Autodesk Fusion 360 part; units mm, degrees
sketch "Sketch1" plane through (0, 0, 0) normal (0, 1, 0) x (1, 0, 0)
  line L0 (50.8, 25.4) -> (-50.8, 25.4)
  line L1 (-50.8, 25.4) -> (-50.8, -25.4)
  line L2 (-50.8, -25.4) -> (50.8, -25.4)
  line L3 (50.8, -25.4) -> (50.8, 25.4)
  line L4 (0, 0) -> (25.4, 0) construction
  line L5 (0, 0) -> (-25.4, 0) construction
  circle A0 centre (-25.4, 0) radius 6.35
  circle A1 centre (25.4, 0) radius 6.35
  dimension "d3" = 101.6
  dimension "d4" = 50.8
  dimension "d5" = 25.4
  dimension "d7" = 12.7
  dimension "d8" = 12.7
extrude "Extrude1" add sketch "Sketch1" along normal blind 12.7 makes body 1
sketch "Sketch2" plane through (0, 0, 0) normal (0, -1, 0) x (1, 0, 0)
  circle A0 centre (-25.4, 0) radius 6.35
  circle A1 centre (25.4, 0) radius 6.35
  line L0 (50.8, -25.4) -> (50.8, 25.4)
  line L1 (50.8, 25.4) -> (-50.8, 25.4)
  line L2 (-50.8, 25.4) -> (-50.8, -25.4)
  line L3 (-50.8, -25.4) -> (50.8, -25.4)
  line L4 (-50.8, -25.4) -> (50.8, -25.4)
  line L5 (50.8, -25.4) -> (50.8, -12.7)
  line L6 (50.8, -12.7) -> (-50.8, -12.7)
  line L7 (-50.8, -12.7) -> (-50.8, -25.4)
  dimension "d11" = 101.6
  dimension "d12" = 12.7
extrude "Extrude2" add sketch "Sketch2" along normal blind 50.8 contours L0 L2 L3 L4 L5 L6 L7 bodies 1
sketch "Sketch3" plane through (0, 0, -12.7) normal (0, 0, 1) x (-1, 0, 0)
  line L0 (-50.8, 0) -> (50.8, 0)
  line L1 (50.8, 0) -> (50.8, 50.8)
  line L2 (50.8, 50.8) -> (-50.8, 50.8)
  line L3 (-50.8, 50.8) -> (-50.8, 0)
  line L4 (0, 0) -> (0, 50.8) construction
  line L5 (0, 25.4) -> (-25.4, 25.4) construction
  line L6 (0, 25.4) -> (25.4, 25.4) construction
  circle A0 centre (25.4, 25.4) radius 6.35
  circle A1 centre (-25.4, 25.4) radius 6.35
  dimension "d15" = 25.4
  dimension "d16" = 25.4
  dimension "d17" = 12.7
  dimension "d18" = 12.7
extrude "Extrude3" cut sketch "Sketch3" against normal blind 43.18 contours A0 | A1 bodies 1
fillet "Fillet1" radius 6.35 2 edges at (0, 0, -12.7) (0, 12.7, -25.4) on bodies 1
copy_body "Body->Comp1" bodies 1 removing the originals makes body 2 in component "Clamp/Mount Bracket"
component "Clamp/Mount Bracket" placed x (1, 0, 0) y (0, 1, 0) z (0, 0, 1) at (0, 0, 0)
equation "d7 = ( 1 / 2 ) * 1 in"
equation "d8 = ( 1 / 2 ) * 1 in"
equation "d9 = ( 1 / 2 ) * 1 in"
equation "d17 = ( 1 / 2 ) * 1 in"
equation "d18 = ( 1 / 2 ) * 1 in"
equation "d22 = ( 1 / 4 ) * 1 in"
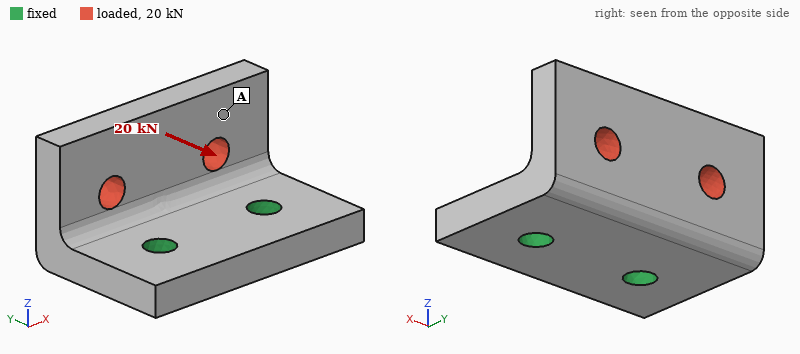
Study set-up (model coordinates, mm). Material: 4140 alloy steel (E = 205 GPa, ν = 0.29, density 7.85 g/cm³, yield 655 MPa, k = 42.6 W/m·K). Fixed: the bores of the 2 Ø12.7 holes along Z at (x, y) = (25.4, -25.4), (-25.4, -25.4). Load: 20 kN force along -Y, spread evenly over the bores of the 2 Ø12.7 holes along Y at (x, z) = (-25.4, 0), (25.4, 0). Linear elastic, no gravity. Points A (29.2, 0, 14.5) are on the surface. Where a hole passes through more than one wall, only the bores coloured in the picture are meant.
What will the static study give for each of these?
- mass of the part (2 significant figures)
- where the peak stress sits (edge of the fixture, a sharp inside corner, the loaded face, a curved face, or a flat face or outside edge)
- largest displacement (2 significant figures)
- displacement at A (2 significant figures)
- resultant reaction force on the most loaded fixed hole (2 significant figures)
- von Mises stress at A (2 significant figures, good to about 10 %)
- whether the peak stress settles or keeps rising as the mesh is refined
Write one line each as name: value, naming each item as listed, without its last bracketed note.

mass of the part: 980 g
where the peak stress sits: edge of the fixture
largest displacement: 0.16 mm
displacement at A: 0.11 mm
resultant reaction force on the most loaded fixed hole: 10 kN
von Mises stress at A: 33 MPa
whether the peak stress settles or keeps rising as the mesh is refined: keeps rising
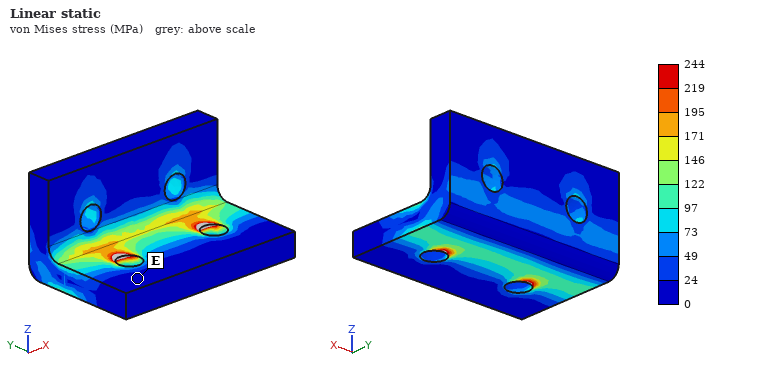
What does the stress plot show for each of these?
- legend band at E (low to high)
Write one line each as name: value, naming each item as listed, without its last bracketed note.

legend band at E: 0 to 24 MPa
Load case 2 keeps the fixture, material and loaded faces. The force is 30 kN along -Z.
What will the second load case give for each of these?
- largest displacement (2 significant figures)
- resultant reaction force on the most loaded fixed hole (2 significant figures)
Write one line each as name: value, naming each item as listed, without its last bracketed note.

largest displacement: 0.21 mm
resultant reaction force on the most loaded fixed hole: 15 kN
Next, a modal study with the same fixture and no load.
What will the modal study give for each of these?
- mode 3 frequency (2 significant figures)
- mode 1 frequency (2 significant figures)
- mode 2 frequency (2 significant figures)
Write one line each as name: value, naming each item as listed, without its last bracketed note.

mode 3 frequency: 6500 Hz
mode 1 frequency: 2600 Hz
mode 2 frequency: 4000 Hz
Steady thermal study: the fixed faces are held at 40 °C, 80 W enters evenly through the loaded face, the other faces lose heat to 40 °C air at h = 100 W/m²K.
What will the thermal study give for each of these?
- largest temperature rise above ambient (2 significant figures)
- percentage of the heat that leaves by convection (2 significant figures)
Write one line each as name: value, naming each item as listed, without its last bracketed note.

largest temperature rise above ambient: 44 K
percentage of the heat that leaves by convection: 52 %
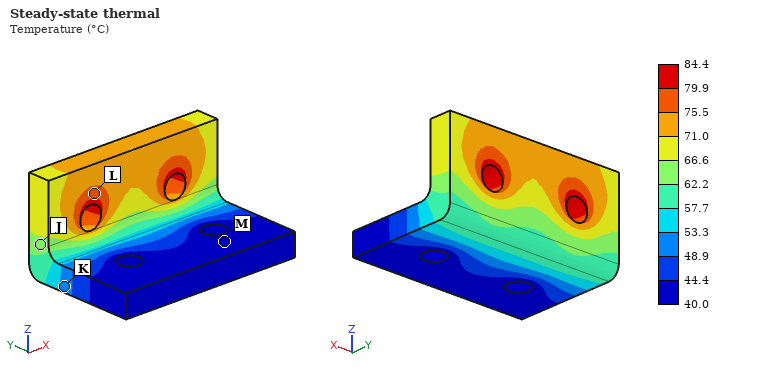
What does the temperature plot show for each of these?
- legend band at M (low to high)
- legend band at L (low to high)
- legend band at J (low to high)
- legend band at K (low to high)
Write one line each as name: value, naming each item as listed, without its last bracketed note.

legend band at M: 40.0 to 44.4 °C
legend band at L: 75.5 to 79.9 °C
legend band at J: 62.2 to 66.6 °C
legend band at K: 48.9 to 53.3 °C
